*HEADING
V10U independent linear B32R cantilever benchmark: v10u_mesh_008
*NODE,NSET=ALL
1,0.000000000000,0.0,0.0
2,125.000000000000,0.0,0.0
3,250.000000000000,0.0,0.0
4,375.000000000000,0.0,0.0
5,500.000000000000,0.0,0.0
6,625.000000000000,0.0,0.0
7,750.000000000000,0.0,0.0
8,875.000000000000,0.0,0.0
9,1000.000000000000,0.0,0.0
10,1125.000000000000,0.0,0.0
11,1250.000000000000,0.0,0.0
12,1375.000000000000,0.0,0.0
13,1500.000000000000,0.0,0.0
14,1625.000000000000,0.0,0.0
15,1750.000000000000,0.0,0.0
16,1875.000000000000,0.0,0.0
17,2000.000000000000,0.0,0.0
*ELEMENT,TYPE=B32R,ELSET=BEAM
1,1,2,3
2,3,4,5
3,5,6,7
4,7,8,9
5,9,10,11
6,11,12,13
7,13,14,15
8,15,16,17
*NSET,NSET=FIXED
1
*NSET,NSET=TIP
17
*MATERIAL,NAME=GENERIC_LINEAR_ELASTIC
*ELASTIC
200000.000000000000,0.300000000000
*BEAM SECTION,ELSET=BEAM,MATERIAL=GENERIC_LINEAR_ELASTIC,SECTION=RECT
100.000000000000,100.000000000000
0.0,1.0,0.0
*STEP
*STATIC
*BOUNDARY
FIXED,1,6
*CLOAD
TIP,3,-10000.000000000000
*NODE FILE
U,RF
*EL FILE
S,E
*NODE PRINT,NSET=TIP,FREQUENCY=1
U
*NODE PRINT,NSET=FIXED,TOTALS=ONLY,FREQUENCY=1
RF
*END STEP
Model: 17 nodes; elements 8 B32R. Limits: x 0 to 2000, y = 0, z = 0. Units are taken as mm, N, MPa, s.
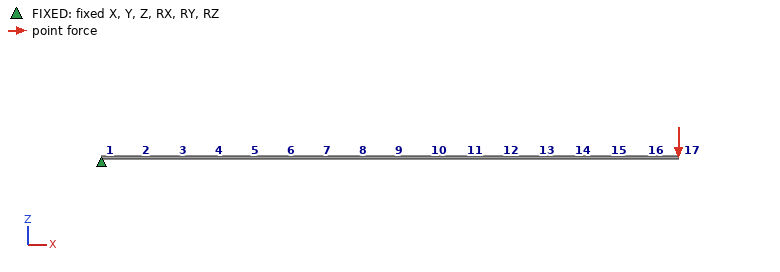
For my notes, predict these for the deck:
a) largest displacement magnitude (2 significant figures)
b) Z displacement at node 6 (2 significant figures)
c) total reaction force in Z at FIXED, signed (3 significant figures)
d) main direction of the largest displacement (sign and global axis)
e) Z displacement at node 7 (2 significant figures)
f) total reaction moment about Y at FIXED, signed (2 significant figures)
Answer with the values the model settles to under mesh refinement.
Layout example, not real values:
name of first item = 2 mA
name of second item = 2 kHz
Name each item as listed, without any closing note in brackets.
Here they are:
largest displacement magnitude = 16 mm
Z displacement at node 6 = -2.1 mm
total reaction force in Z at FIXED, signed = 10000 N
main direction of the largest displacement = -Z
Z displacement at node 7 = -3.0 mm
total reaction moment about Y at FIXED, signed = -2.0e+07 N·mm
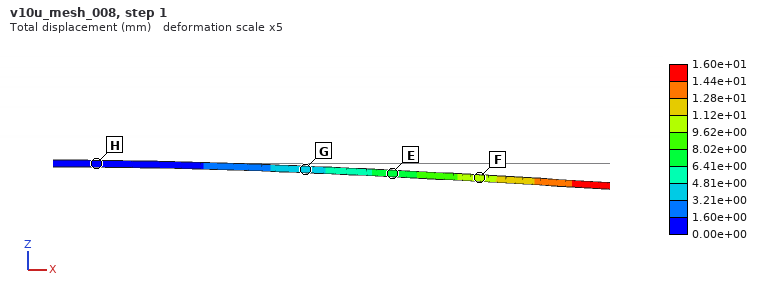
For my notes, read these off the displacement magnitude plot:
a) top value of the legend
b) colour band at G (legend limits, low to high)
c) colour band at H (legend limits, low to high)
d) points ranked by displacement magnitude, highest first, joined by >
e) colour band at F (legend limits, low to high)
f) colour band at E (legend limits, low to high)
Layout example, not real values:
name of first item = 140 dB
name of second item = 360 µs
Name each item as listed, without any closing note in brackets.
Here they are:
top value of the legend = 1.60e+01 mm
colour band at G = 3.21e+00 to 4.81e+00 mm
colour band at H = 0.00e+00 to 1.60e+00 mm
points ranked by displacement magnitude, highest first, joined by > = F > E > G > H
colour band at F = 9.62e+00 to 1.12e+01 mm
colour band at E = 6.41e+00 to 8.02e+00 mm
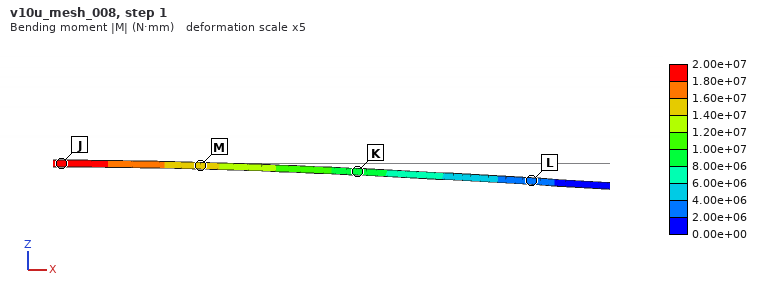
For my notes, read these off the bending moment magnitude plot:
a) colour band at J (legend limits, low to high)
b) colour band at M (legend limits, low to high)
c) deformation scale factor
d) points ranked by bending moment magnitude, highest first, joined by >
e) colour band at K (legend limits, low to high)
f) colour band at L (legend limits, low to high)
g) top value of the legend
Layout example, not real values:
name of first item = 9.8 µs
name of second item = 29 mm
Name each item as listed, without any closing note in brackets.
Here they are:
colour band at J = 1.80e+07 to 2.00e+07 N·mm
colour band at M = 1.40e+07 to 1.60e+07 N·mm
deformation scale factor = 5
points ranked by bending moment magnitude, highest first, joined by > = J > M > K > L
colour band at K = 8.00e+06 to 1.00e+07 N·mm
colour band at L = 2.00e+06 to 4.00e+06 N·mm
top value of the legend = 2.00e+07 N·mm
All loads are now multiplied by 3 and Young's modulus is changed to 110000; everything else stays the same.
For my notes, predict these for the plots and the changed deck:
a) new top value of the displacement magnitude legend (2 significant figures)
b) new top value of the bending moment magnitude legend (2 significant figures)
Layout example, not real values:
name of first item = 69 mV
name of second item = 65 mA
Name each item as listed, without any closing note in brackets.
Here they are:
new top value of the displacement magnitude legend = 87 mm
new top value of the bending moment magnitude legend = 6.0e+07 N·mm
